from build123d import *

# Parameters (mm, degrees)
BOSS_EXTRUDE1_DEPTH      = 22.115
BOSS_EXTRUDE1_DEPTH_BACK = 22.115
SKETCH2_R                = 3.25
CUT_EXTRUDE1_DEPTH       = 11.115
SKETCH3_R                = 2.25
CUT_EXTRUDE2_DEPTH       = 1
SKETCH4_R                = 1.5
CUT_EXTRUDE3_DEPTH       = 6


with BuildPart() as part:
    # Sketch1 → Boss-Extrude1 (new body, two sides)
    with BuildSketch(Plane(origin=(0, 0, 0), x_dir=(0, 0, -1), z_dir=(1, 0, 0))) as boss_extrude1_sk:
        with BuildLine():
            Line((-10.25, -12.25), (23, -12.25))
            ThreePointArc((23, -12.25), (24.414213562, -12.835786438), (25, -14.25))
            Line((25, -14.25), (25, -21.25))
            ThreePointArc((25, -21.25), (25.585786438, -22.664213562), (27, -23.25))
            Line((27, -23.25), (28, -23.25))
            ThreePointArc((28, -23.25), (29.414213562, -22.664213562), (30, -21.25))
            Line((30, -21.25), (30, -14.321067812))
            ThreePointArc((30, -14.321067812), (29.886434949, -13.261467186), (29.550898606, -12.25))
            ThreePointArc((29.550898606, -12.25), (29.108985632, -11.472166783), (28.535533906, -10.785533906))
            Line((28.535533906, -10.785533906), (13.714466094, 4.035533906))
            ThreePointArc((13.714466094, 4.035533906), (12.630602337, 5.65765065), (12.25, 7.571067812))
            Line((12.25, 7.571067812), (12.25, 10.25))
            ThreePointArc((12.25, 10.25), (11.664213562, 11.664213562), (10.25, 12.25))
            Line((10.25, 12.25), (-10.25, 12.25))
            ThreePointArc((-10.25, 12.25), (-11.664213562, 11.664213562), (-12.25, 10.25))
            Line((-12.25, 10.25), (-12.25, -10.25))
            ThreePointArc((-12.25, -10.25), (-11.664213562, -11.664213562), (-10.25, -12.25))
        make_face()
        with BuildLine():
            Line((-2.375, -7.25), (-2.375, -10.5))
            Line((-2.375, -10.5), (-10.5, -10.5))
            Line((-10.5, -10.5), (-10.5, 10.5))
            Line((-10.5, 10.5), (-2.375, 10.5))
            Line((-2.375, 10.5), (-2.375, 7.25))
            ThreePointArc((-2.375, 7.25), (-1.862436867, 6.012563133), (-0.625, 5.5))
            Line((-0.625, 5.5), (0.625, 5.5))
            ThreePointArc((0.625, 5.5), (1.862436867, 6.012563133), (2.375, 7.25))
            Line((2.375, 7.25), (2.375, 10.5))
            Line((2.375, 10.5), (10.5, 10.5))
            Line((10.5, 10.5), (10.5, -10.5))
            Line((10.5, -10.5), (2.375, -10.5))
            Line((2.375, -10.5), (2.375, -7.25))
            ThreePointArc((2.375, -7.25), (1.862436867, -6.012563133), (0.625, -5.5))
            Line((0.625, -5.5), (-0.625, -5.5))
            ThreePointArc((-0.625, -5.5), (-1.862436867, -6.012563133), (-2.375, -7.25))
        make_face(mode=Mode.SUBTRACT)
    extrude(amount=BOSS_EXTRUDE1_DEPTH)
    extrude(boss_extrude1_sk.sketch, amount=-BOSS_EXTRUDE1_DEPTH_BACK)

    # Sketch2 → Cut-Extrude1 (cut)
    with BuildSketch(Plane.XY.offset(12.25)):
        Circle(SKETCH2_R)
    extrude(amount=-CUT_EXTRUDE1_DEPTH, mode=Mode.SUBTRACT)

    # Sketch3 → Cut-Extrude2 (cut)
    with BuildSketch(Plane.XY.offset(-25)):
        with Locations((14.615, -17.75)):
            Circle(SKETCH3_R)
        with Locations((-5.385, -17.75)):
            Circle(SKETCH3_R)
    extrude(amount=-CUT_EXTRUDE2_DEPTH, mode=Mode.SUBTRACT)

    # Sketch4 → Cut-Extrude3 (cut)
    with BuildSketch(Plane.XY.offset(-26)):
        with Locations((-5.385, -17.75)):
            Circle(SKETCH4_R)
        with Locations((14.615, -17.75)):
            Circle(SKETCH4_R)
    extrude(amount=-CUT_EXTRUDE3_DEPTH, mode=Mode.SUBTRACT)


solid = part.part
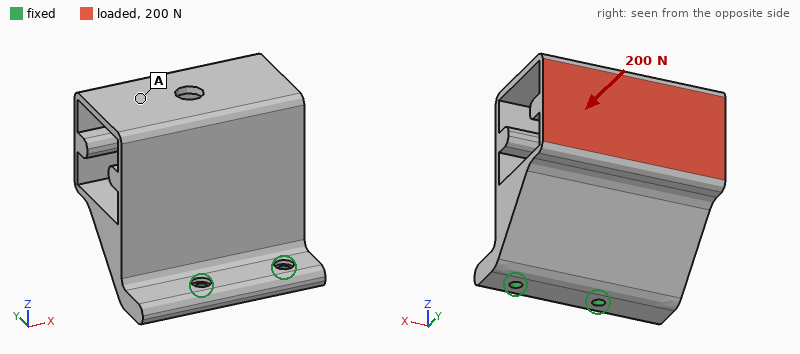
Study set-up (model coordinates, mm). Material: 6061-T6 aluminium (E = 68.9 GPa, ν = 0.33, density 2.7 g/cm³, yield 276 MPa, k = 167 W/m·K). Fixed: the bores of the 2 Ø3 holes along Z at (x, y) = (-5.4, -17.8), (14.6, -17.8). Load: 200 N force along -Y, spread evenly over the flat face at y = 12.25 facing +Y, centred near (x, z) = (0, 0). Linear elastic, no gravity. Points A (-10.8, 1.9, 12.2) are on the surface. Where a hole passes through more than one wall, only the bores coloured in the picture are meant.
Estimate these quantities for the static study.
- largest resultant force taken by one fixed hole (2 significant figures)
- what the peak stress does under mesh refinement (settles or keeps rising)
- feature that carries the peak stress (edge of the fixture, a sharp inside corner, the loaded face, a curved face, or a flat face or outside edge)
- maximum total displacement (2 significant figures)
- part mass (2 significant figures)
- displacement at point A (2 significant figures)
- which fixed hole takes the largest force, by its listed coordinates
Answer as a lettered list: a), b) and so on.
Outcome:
a) 140 N
b) keeps rising
c) edge of the fixture
d) 0.20 mm
e) 49 g
f) 0.19 mm
g) (-5.4, -17.8)
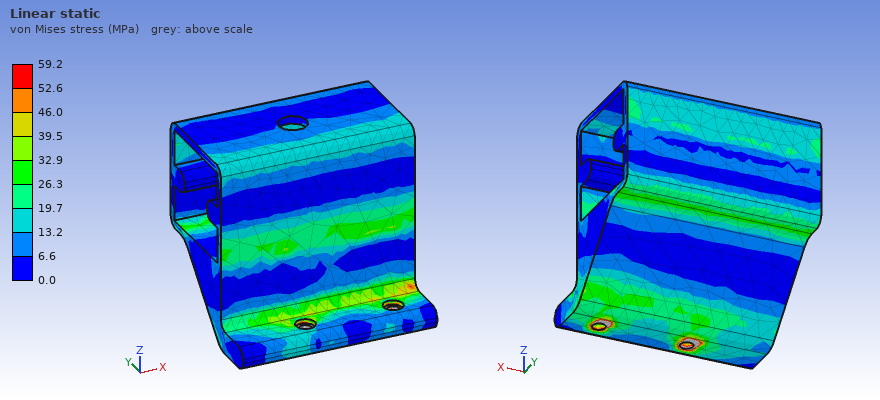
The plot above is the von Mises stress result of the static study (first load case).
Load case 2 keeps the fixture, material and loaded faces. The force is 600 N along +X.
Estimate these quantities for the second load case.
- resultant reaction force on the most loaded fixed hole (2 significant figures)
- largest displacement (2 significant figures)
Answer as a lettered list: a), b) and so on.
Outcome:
a) 1.2 kN
b) 78 µm
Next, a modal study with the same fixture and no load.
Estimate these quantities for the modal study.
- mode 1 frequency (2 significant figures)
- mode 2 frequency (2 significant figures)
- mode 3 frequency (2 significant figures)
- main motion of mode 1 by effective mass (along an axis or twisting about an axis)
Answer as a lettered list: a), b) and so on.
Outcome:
a) 1100 Hz
b) 3500 Hz
c) 3800 Hz
d) along Y
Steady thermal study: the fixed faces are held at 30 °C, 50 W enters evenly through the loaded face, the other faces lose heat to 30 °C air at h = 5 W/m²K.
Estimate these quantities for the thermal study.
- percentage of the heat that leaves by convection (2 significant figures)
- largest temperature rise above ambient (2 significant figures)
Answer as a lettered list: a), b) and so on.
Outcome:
a) 4.1 %
b) 73 K
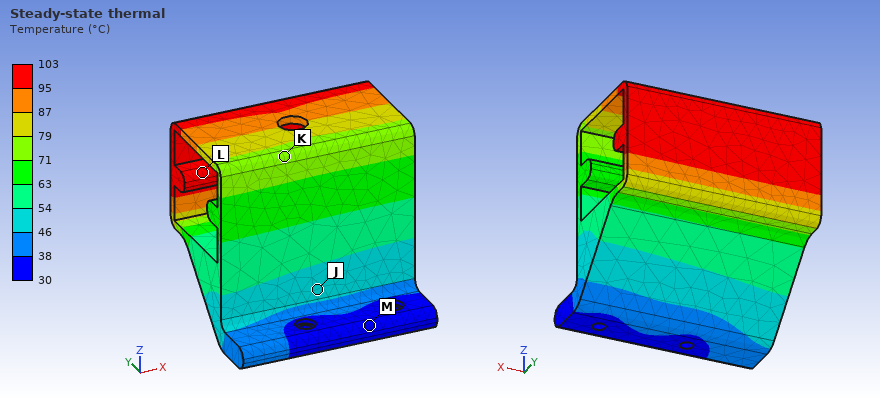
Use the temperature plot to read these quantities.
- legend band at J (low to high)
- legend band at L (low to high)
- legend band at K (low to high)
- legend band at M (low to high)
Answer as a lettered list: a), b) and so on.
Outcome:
a) 46 to 54 °C
b) 95 to 103 °C
c) 71 to 79 °C
d) 30 to 38 °C
